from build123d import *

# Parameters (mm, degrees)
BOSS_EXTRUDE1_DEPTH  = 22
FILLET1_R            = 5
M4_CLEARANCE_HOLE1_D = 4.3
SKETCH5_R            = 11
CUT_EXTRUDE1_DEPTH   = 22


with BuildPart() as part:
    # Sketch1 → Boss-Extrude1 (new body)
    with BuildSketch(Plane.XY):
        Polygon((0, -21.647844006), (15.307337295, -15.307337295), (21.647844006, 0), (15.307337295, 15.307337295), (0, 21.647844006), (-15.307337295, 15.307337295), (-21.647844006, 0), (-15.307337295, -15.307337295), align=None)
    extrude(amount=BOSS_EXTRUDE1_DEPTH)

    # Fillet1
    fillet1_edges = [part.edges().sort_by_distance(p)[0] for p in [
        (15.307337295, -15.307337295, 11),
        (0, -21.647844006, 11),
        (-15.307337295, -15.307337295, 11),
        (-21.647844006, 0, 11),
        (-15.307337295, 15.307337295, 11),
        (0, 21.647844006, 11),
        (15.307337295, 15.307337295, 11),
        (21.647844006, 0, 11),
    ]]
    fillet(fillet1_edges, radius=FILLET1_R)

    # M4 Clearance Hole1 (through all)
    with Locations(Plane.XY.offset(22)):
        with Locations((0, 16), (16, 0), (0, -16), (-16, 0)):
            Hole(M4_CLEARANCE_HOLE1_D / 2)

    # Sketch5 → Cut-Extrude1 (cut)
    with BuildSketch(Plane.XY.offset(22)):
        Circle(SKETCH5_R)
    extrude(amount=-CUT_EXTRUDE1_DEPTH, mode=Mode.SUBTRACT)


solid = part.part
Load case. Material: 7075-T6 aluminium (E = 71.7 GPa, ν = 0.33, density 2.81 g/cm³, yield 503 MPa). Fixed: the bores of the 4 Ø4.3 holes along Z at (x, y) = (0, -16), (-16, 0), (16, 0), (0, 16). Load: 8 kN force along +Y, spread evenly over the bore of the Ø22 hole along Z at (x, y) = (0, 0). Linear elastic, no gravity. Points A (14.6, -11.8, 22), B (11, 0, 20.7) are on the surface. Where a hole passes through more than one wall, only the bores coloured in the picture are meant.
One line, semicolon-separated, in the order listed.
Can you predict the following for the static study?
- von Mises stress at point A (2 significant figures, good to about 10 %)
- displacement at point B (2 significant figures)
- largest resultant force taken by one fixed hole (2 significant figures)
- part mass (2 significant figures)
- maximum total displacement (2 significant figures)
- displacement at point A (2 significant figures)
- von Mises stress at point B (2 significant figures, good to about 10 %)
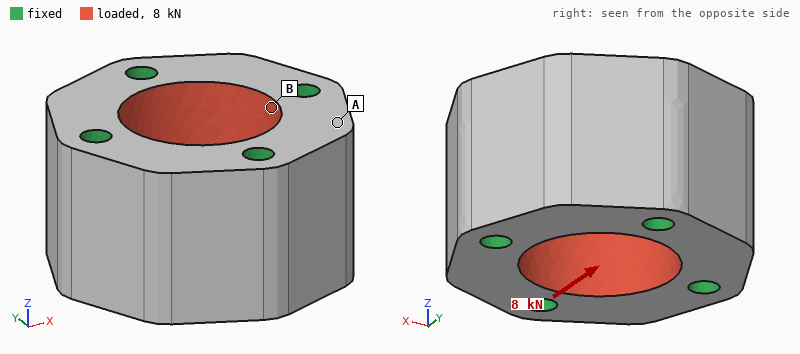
4.1 MPa; 1.0 µm; 2.2 kN; 55 g; 1.5 µm; 1.0 µm; 9.2 MPa
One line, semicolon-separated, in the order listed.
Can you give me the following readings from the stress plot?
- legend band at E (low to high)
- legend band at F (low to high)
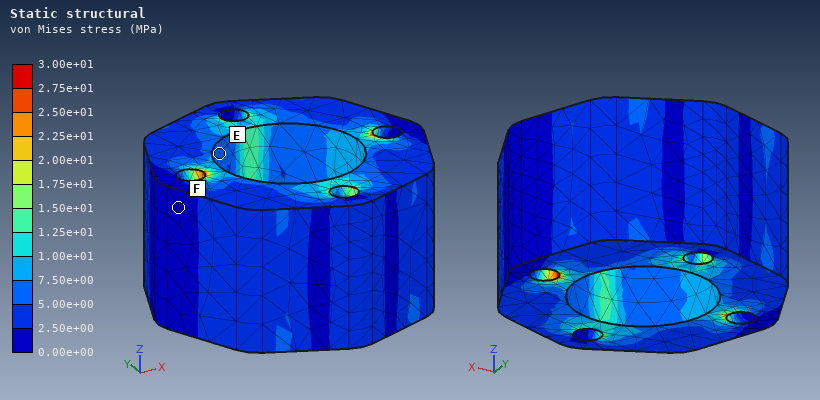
5.00e+00 to 7.50e+00 MPa; 0.00e+00 to 2.50e+00 MPa
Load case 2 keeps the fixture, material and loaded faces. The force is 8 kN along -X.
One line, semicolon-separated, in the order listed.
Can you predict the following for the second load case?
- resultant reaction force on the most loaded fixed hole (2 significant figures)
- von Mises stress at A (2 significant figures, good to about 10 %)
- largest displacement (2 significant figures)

2.2 kN; 4.1 MPa; 1.5 µm
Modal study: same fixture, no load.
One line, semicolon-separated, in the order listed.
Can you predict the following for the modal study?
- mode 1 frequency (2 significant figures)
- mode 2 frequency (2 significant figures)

54 kHz; 56 kHz
